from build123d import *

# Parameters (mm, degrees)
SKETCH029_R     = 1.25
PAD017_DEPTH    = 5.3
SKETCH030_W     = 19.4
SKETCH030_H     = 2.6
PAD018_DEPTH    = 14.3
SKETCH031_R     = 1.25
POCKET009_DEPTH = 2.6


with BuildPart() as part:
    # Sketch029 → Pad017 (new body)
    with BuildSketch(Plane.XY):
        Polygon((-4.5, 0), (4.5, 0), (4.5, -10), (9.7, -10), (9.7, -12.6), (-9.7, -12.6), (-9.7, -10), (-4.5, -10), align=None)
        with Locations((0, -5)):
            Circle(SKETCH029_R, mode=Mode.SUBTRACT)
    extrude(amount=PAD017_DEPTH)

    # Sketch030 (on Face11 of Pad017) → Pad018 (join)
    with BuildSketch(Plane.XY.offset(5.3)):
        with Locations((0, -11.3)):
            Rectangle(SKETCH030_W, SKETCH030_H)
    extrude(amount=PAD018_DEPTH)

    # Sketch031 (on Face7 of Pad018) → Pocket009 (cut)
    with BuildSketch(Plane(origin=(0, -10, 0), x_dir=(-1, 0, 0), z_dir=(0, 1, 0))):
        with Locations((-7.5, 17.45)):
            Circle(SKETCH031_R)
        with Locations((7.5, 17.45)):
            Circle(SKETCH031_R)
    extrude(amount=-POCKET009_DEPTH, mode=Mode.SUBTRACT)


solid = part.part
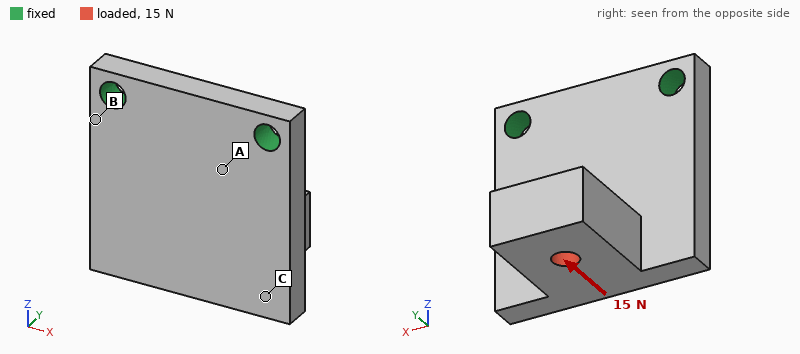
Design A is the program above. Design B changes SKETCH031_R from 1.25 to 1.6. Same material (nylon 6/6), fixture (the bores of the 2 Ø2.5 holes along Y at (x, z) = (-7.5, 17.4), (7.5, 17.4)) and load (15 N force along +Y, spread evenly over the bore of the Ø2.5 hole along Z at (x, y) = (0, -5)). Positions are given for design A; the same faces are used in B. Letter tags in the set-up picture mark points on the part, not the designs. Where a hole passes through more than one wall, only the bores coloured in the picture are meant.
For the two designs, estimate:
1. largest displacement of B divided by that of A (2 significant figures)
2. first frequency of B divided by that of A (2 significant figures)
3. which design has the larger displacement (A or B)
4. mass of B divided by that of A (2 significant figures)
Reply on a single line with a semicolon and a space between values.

0.90; 1.1; A; 0.99
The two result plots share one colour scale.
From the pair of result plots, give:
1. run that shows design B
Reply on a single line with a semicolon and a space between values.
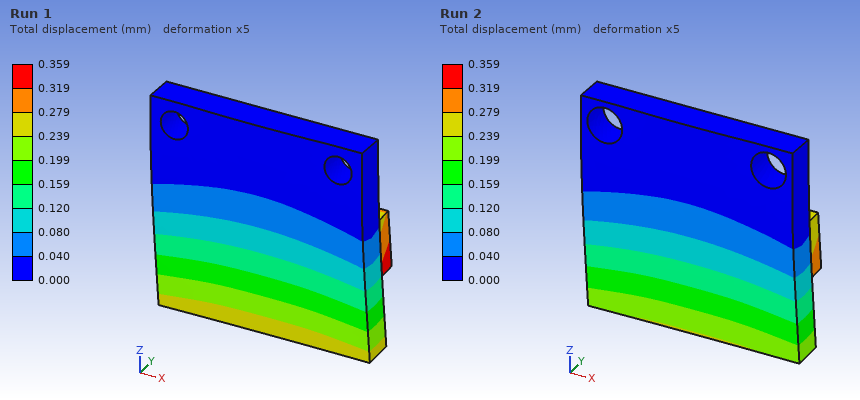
Run 2
